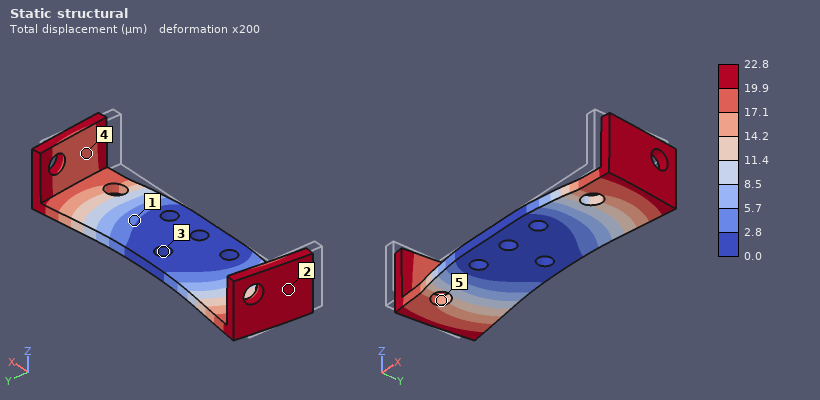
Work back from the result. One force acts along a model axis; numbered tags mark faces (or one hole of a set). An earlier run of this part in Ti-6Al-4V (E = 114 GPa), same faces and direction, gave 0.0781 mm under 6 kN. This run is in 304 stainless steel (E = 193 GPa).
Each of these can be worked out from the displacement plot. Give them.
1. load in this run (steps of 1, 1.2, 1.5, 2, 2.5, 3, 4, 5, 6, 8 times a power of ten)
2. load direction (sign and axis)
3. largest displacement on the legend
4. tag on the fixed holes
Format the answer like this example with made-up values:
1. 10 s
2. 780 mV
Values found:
1. 3 kN
2. +Y
3. 22.8 µm
4. 3
